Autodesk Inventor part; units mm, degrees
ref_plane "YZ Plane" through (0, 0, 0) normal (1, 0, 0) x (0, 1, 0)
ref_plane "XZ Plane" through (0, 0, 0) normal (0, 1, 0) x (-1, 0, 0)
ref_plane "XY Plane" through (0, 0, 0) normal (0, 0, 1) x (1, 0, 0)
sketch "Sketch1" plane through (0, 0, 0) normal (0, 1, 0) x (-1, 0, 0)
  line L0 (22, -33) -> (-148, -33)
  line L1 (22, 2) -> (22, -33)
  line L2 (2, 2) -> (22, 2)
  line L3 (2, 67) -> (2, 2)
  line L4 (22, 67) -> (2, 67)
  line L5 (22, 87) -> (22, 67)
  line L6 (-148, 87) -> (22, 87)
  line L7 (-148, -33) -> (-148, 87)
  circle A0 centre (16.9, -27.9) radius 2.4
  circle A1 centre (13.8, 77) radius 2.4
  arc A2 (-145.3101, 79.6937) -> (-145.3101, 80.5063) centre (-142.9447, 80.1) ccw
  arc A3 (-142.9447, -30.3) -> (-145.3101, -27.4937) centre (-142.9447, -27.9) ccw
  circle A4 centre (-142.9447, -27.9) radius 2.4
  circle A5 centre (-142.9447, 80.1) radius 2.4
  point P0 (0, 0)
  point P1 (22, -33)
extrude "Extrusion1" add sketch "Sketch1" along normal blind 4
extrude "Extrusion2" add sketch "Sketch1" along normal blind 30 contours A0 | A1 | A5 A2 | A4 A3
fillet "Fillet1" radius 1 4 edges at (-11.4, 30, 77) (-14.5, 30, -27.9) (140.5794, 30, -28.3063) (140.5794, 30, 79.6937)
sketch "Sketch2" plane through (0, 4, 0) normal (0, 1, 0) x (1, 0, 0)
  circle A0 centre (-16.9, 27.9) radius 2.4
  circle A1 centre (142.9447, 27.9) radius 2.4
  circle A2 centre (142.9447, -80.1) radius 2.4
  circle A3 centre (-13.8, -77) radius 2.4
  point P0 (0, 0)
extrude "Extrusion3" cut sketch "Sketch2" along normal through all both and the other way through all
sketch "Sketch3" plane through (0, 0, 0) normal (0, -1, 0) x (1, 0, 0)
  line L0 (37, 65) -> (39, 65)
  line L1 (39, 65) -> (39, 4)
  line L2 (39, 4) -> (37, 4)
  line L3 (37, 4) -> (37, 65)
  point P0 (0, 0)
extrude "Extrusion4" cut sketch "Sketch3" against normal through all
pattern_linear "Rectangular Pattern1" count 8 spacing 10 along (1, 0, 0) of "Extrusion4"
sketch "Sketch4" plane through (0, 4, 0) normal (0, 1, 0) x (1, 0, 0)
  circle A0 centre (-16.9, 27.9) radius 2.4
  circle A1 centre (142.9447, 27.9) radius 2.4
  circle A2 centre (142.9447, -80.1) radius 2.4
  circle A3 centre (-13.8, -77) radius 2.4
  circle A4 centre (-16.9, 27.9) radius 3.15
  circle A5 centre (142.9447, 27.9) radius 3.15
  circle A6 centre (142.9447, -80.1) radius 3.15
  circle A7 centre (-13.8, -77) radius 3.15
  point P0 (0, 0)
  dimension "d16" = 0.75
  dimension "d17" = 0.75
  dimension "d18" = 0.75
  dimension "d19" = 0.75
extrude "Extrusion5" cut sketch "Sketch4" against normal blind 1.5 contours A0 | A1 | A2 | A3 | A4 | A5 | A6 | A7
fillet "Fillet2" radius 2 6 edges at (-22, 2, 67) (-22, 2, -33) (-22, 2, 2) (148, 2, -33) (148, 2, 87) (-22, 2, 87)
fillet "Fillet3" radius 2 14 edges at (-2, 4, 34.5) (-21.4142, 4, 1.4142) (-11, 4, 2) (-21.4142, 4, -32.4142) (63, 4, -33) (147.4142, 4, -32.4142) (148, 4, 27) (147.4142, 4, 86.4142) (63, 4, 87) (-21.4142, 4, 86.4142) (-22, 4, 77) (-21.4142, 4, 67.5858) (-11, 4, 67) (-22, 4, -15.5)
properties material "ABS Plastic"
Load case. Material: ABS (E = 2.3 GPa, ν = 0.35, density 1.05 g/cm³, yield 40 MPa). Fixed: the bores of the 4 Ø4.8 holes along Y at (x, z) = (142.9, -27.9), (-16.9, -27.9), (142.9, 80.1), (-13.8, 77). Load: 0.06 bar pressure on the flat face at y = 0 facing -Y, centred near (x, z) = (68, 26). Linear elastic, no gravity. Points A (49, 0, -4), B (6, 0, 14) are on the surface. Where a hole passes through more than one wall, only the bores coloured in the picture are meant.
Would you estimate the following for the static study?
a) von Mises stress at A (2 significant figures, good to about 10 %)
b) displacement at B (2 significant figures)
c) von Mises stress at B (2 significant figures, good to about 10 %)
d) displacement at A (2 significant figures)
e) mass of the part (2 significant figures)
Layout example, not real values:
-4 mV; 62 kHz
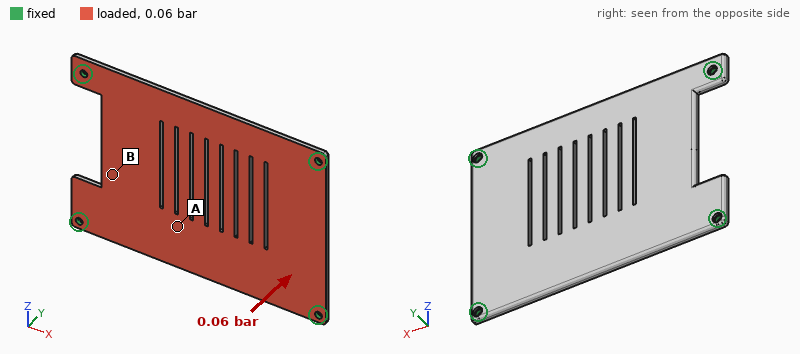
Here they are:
4.0 MPa; 0.89 mm; 1.8 MPa; 2.0 mm; 75 g
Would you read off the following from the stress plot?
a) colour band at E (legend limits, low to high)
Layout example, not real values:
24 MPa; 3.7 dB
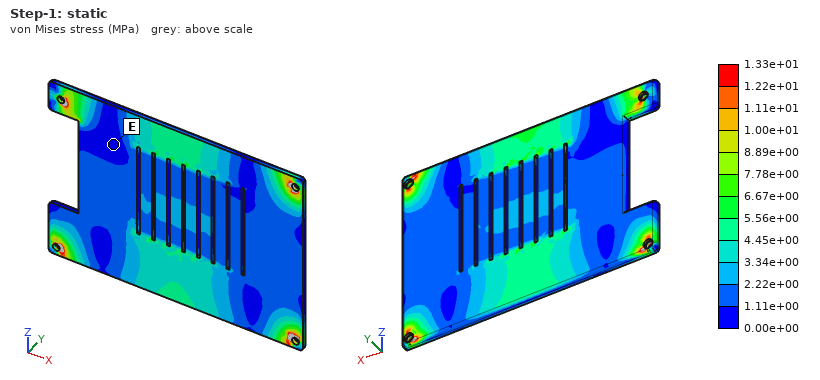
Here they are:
0.00e+00 to 1.11e+00 MPa
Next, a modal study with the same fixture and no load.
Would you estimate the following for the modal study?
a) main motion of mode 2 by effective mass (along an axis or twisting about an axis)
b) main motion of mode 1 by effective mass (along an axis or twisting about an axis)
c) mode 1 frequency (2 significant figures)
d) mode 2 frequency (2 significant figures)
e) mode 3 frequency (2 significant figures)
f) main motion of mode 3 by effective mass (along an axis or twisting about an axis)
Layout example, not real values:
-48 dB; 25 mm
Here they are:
twisting about X; along Y; 150 Hz; 280 Hz; 350 Hz; twisting about Z
